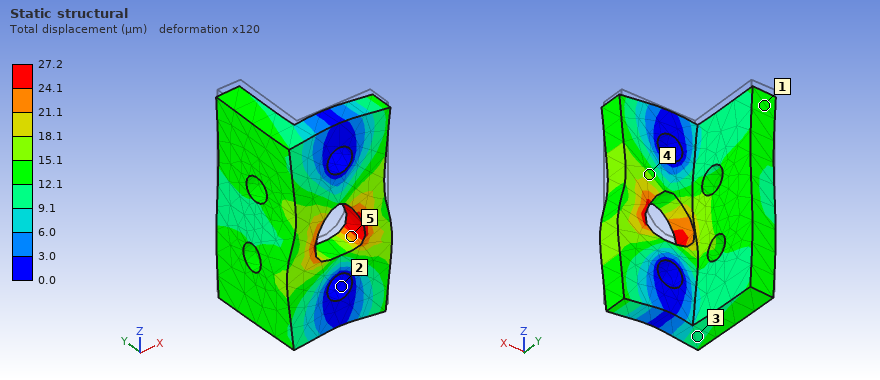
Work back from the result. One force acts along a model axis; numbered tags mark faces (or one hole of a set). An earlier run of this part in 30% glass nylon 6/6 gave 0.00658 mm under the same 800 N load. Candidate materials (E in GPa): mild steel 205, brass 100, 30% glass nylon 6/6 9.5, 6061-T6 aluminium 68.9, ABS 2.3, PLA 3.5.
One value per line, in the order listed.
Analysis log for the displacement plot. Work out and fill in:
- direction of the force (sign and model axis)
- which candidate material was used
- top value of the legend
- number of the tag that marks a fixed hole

-Z
ABS
27.2 µm
2
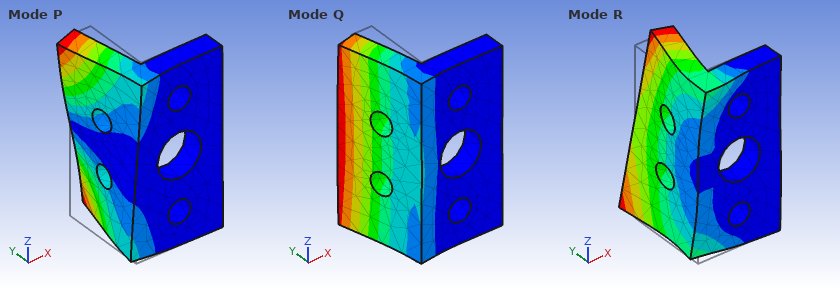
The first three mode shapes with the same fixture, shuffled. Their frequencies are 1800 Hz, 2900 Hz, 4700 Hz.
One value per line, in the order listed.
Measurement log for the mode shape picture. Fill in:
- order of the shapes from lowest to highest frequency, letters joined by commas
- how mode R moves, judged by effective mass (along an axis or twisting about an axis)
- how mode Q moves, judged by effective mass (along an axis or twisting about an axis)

Q, P, R
along Z
along X
